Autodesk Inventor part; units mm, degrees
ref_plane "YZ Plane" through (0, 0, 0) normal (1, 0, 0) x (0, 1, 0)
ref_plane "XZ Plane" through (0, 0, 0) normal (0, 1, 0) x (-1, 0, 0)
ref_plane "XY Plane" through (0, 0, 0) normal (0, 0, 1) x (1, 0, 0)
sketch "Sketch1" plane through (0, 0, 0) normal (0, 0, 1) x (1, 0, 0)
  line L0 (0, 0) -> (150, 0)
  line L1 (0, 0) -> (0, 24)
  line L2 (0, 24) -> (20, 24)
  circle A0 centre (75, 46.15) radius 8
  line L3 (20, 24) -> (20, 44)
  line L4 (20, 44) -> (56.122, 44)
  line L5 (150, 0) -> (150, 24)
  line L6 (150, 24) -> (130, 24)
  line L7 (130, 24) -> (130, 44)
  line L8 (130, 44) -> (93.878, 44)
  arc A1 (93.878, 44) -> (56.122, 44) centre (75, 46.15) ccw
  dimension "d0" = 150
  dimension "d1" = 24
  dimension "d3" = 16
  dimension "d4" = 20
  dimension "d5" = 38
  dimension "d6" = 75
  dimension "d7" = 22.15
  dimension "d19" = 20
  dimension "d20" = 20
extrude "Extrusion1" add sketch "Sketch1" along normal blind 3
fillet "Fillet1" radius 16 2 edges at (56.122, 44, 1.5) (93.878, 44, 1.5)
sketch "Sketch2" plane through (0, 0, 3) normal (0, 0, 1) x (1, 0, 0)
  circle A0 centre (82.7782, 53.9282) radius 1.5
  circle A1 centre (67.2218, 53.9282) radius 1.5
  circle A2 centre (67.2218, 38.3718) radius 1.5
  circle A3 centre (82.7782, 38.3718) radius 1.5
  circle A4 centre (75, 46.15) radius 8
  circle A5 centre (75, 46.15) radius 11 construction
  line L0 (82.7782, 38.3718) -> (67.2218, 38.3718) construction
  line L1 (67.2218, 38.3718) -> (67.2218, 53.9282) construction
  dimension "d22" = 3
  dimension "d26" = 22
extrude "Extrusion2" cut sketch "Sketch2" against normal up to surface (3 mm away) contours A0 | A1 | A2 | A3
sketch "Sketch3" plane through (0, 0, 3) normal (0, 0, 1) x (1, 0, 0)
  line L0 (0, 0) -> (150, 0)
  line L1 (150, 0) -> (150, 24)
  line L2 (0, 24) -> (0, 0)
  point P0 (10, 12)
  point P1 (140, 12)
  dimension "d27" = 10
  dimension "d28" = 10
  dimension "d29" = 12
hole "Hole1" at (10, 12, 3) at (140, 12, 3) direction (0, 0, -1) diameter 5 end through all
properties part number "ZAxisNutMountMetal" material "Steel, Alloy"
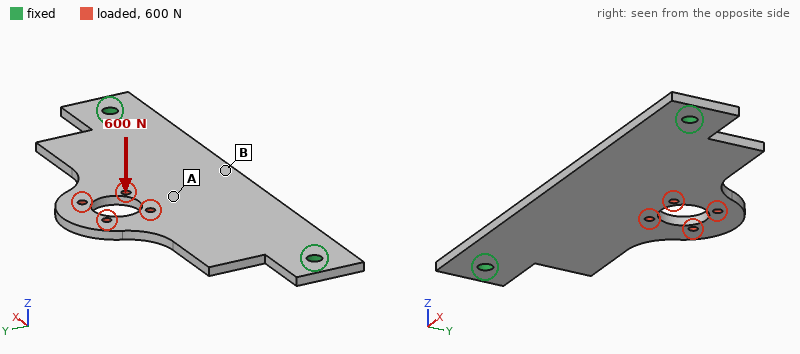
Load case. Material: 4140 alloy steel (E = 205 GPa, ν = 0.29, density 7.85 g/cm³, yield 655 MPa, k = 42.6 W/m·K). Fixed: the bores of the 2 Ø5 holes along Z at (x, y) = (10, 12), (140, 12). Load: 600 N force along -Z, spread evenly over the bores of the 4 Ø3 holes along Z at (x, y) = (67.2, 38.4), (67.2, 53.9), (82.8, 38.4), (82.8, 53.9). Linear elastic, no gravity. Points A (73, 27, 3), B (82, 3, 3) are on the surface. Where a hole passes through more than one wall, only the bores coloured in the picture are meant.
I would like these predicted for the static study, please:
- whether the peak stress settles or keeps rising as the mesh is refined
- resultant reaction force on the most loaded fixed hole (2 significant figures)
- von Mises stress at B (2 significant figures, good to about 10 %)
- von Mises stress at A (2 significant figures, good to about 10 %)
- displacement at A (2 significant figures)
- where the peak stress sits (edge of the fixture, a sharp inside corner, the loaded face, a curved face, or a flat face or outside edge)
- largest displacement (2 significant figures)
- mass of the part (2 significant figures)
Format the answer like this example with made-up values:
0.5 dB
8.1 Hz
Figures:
keeps rising
300 N
80 MPa
160 MPa
0.64 mm
edge of the fixture
1.6 mm
150 g
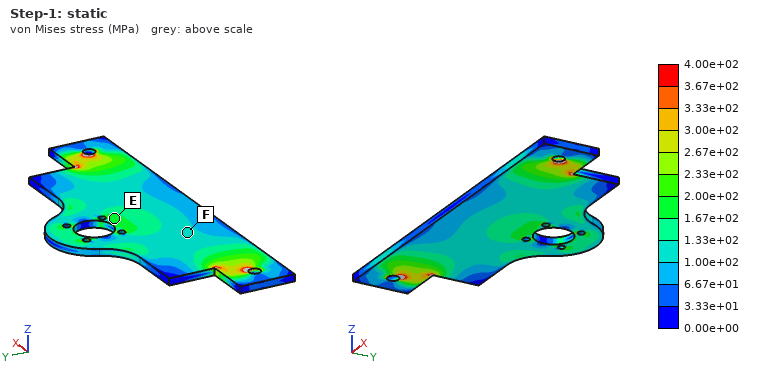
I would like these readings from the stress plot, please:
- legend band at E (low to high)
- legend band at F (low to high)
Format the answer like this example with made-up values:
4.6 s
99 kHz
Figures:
1.67e+02 to 2.00e+02 MPa
1.00e+02 to 1.33e+02 MPa
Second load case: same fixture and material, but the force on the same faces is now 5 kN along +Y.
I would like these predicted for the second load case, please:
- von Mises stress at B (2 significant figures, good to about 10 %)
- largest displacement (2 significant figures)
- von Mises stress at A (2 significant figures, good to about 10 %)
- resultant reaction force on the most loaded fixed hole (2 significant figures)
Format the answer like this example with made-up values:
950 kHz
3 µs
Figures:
58 MPa
47 µm
30 MPa
3.3 kN
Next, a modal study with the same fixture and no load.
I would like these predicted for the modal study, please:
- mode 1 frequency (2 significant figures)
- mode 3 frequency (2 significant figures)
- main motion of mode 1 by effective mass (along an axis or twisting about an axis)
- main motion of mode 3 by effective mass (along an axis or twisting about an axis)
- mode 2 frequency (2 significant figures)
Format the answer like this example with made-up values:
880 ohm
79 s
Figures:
610 Hz
1900 Hz
along Z
twisting about Y
1200 Hz
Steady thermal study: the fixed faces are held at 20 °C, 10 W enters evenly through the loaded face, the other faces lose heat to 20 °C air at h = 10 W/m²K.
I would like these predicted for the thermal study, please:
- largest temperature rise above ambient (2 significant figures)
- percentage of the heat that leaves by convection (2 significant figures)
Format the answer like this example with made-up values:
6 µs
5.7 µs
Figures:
76 K
42 %
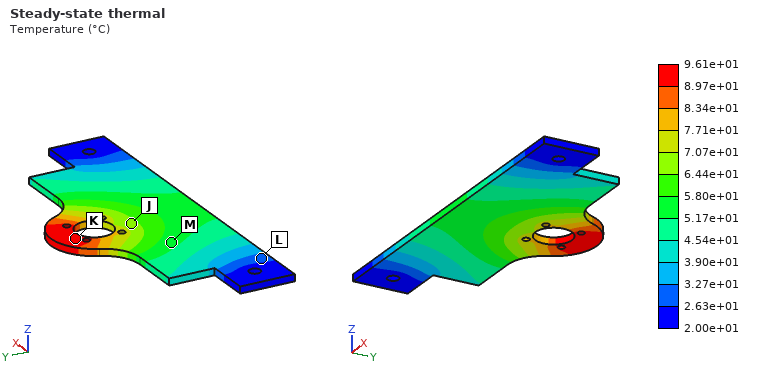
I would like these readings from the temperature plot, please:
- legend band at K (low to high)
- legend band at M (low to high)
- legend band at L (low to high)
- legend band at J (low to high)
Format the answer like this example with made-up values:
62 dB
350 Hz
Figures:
8.97e+01 to 9.61e+01 °C
5.17e+01 to 5.80e+01 °C
2.63e+01 to 3.27e+01 °C
6.44e+01 to 7.07e+01 °C
